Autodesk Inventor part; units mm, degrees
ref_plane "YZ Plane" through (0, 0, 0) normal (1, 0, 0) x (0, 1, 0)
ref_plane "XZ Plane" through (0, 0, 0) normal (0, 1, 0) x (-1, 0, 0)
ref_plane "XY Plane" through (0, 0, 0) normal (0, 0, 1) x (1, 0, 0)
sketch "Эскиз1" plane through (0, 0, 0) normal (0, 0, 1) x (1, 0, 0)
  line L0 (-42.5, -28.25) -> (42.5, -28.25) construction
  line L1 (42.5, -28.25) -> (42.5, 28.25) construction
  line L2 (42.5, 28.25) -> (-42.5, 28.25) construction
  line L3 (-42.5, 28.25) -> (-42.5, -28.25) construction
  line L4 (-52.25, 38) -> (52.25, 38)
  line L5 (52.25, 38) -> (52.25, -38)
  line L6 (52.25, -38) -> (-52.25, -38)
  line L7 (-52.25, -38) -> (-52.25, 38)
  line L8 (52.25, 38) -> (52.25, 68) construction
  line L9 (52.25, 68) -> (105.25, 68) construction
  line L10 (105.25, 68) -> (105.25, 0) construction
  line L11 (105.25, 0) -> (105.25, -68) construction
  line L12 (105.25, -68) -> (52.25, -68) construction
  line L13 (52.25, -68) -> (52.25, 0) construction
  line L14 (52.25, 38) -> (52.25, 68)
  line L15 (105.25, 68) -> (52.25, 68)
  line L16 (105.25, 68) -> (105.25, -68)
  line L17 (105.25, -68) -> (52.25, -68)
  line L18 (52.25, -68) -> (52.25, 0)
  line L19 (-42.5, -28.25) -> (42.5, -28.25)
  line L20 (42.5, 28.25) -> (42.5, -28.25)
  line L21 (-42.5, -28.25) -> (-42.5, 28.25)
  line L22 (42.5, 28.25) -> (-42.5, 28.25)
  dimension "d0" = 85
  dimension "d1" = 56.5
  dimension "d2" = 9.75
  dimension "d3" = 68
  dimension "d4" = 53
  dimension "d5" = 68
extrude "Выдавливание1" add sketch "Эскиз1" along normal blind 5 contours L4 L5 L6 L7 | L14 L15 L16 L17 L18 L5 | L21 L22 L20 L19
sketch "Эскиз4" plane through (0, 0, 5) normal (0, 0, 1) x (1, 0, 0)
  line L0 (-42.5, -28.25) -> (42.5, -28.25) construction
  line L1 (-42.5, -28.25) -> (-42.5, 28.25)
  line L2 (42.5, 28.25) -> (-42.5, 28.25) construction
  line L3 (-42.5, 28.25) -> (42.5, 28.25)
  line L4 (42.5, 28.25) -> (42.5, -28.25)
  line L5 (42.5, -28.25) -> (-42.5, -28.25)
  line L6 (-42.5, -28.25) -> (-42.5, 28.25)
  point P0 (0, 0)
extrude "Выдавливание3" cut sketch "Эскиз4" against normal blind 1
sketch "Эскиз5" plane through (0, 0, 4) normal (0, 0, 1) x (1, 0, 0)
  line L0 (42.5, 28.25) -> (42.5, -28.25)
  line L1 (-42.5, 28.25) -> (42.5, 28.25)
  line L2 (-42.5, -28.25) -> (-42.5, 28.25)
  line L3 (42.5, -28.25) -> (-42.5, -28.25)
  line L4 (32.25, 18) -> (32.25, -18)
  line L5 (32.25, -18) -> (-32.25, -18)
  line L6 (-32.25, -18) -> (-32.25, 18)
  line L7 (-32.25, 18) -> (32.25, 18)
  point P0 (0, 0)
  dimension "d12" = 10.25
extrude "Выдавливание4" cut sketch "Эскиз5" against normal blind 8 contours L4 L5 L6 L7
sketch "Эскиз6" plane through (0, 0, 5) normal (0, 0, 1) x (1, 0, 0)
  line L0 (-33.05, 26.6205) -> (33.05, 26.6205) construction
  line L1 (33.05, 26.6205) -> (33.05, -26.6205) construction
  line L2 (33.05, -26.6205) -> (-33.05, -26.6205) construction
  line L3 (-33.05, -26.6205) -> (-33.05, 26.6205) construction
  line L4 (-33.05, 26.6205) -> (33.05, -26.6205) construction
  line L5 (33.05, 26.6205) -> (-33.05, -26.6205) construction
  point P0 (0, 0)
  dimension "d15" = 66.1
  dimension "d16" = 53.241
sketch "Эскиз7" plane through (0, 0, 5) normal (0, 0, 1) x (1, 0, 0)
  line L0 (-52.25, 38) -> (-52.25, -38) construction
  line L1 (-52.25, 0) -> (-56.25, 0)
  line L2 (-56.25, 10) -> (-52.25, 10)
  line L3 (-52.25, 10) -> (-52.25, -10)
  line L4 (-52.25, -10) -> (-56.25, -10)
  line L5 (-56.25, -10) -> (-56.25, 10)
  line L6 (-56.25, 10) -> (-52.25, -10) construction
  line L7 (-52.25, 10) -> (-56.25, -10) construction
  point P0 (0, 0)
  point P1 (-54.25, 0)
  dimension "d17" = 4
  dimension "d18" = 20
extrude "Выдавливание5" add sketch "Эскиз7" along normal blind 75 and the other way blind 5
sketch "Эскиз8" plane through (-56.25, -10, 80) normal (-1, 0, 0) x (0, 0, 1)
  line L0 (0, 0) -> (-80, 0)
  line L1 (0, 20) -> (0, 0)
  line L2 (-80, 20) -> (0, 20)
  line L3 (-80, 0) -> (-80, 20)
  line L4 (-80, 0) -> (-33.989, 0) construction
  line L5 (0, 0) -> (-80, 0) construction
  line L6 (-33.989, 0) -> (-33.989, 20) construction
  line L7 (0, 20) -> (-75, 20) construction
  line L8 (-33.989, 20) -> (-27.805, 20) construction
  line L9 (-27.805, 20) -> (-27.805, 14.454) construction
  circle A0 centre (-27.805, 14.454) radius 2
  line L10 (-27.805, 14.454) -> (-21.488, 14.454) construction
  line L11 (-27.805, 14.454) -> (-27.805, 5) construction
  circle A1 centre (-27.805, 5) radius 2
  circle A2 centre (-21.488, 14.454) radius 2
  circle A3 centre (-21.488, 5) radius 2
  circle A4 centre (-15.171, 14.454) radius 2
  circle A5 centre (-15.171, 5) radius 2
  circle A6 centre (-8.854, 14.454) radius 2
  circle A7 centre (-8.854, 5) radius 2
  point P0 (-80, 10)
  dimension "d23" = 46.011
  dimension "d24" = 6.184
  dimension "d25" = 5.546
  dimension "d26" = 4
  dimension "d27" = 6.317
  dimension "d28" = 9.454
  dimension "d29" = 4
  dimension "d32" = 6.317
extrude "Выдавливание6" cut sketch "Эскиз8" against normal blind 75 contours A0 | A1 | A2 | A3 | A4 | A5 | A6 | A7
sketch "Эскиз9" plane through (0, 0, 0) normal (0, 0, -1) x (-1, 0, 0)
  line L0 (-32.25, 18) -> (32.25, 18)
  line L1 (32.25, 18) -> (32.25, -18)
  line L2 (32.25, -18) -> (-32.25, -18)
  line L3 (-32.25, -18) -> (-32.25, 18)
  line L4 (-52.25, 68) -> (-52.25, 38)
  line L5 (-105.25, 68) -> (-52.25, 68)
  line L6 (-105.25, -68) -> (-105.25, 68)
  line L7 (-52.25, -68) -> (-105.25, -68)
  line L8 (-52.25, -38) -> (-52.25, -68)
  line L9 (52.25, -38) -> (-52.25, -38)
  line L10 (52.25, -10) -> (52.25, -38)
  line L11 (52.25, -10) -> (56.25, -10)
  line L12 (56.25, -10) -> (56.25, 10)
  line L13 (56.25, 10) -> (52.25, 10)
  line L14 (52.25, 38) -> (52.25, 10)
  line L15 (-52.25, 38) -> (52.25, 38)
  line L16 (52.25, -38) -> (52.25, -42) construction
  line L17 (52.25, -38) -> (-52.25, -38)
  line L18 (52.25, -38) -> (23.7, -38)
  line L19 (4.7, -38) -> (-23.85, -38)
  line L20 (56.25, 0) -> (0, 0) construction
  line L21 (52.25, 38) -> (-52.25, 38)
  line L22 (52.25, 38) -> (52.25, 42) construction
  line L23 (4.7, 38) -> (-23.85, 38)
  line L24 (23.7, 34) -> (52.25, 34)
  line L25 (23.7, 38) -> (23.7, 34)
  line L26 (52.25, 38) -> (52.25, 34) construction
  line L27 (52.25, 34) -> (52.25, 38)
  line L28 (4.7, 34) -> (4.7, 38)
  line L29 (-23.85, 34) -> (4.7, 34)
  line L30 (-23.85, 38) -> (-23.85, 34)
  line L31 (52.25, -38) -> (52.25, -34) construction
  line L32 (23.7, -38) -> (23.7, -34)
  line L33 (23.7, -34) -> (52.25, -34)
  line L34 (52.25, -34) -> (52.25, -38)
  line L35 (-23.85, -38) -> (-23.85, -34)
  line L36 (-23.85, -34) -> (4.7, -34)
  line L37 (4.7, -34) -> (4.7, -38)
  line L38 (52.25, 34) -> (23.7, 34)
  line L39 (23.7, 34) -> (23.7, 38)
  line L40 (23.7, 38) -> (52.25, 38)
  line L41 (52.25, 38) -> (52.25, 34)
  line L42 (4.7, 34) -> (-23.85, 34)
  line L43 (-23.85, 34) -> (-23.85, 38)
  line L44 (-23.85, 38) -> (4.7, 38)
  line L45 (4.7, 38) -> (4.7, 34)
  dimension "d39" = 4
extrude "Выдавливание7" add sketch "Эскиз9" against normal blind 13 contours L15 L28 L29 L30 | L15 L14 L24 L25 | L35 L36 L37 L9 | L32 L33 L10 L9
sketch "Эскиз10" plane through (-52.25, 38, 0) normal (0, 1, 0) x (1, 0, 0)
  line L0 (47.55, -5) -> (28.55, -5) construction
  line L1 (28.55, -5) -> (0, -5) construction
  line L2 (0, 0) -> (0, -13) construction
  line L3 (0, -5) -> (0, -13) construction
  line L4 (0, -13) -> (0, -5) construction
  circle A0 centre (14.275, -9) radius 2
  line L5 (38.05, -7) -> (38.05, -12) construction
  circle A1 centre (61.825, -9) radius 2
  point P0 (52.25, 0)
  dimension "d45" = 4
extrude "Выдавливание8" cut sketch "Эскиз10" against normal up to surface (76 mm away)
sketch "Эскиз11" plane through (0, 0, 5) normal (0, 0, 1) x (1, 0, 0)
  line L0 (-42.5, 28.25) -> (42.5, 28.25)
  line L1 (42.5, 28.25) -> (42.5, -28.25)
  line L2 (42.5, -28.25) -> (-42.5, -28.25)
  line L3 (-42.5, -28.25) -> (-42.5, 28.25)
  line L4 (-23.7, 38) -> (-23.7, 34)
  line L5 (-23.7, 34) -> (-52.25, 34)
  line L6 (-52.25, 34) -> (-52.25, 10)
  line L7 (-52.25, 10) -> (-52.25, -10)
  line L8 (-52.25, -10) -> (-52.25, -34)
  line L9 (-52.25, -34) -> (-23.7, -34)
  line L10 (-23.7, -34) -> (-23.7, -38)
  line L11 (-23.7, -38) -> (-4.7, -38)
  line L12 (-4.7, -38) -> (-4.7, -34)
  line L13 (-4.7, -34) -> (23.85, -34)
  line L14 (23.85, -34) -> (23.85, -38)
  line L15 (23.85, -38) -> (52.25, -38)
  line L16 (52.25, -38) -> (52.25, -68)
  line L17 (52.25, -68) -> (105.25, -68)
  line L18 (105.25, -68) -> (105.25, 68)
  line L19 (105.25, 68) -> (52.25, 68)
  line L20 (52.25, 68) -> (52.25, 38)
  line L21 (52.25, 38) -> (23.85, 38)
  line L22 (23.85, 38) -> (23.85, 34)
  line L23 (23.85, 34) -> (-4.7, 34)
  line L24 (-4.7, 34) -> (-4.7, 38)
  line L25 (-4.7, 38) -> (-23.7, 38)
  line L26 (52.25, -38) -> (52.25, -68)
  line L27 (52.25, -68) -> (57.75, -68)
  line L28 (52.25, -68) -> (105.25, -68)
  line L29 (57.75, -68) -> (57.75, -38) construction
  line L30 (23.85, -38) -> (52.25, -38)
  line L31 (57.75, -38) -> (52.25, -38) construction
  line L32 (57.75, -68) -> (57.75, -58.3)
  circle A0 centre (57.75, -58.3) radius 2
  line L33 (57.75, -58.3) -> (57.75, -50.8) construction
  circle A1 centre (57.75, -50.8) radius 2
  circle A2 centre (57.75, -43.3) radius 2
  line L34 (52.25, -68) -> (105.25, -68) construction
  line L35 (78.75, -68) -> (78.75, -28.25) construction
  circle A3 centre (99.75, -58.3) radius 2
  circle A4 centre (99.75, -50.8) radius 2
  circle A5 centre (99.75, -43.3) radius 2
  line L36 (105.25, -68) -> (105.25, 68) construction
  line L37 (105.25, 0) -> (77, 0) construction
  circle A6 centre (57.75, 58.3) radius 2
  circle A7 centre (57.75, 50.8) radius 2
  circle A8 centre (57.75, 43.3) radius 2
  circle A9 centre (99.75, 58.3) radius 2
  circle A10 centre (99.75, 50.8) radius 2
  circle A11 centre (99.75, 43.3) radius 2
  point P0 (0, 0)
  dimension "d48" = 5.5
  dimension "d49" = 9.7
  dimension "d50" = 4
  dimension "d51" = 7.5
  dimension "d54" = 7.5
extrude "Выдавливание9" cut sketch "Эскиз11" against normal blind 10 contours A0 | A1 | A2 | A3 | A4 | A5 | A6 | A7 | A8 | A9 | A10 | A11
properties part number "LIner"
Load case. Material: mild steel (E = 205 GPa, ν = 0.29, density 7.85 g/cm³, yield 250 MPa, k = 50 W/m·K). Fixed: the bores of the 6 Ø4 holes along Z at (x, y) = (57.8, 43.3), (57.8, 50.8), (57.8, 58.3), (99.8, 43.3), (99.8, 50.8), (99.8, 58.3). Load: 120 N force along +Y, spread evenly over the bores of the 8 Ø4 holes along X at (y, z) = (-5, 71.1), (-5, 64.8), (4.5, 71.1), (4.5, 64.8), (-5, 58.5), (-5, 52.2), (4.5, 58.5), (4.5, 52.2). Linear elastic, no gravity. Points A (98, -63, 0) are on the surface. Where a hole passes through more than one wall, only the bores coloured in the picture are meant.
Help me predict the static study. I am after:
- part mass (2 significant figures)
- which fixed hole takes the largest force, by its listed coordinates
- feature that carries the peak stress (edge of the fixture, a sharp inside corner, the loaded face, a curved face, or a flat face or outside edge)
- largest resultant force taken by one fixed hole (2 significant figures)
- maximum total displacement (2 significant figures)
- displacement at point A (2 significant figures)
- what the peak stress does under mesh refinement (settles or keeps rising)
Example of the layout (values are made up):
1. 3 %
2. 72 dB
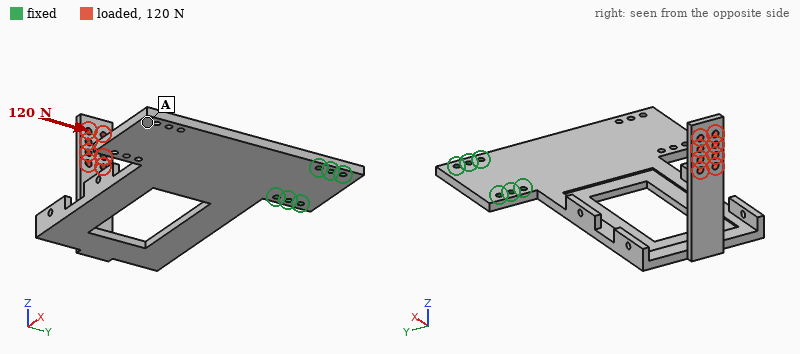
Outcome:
1. 550 g
2. (57.8, 43.3)
3. edge of the fixture
4. 410 N
5. 0.80 mm
6. 0.16 mm
7. keeps rising
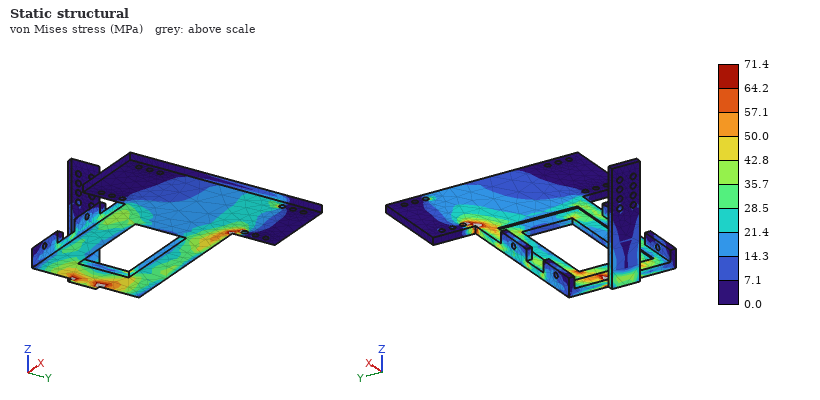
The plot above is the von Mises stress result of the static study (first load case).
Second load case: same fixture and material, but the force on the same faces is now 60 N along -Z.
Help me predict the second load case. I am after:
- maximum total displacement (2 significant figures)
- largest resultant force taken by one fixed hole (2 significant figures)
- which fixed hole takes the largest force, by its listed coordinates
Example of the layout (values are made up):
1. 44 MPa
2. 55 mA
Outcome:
1. 0.58 mm
2. 280 N
3. (57.8, 43.3)
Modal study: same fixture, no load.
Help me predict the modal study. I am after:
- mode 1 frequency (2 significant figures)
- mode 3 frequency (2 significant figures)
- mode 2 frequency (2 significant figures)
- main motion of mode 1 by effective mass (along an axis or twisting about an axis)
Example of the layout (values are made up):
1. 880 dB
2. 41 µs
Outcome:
1. 170 Hz
2. 470 Hz
3. 280 Hz
4. along Z
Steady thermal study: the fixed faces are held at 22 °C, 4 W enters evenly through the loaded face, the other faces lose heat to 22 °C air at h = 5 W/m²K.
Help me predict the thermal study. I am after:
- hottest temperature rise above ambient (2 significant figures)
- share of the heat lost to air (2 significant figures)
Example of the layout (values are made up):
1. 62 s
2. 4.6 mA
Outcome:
1. 82 K
2. 62 %
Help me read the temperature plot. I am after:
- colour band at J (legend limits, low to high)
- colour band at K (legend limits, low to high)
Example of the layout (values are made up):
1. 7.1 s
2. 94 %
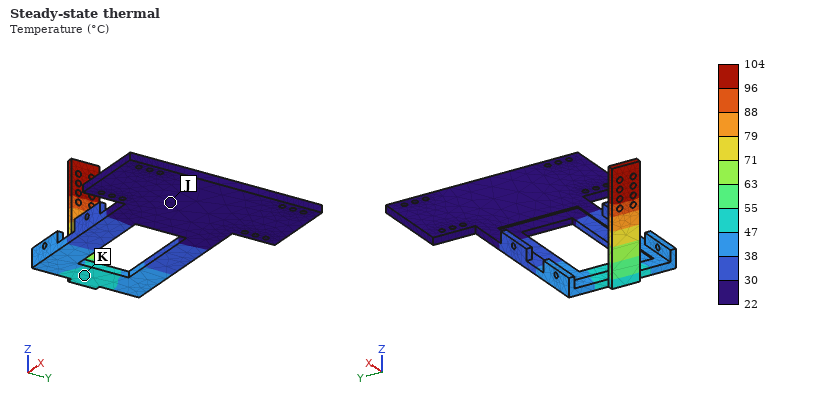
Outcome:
1. 22 to 30 °C
2. 47 to 55 °C
